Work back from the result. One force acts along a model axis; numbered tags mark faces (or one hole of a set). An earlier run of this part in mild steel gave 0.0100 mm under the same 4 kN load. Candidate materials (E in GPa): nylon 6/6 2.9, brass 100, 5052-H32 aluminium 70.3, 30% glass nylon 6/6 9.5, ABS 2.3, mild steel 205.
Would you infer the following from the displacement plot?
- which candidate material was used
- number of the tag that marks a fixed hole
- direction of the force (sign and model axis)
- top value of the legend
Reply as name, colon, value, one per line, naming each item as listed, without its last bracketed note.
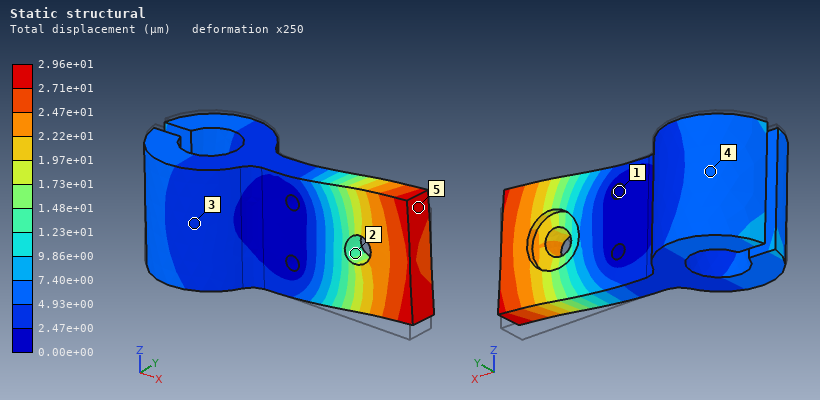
which candidate material was used: 5052-H32 aluminium
number of the tag that marks a fixed hole: 1
direction of the force: +Z
top value of the legend: 2.96e+01 µm
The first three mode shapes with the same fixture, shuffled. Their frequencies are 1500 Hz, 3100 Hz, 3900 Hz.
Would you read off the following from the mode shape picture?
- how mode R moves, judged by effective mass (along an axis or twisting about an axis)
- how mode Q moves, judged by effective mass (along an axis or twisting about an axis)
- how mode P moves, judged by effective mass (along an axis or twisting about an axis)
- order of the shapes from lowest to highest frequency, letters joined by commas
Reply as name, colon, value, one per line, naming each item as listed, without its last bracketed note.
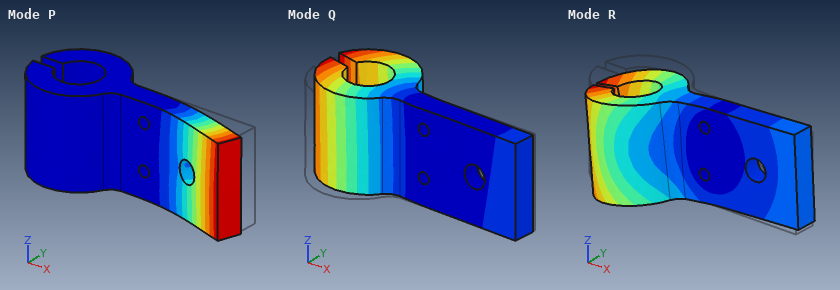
how mode R moves, judged by effective mass: along Z
how mode Q moves, judged by effective mass: along Y
how mode P moves, judged by effective mass: along Y
order of the shapes from lowest to highest frequency, letters joined by commas: Q, P, R
